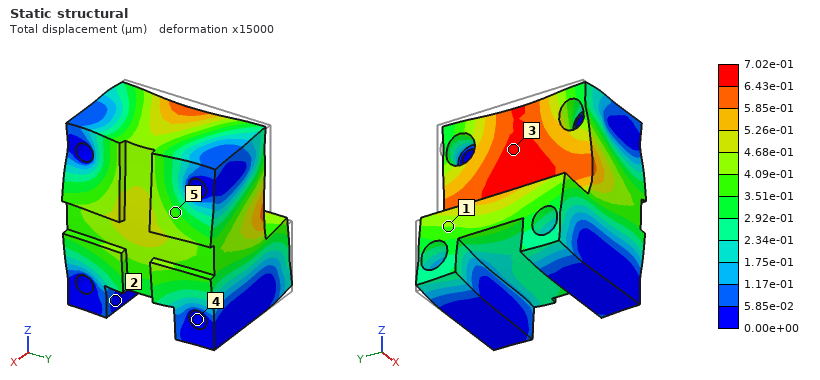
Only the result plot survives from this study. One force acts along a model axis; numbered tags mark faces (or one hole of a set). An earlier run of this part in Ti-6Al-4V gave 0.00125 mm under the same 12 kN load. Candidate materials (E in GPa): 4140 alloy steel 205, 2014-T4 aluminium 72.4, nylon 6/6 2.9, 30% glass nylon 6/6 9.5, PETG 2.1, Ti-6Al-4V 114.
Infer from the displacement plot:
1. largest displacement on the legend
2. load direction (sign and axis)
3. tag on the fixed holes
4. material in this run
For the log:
7.02e-01 µm
+X
4
4140 alloy steel
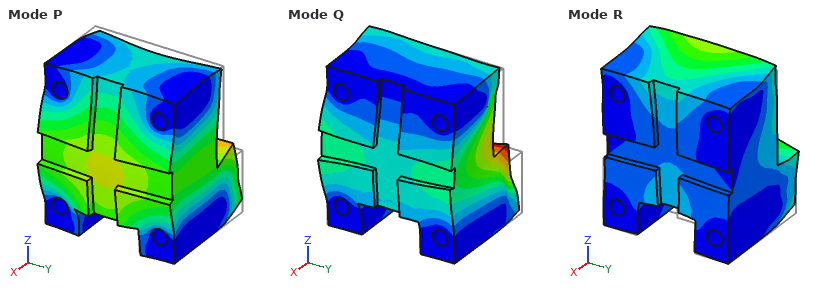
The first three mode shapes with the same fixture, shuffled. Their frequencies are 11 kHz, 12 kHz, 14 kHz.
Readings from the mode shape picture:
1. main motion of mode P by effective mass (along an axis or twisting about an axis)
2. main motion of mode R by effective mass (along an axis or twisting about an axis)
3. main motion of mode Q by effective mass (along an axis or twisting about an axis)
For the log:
along X
along Z
along Y
